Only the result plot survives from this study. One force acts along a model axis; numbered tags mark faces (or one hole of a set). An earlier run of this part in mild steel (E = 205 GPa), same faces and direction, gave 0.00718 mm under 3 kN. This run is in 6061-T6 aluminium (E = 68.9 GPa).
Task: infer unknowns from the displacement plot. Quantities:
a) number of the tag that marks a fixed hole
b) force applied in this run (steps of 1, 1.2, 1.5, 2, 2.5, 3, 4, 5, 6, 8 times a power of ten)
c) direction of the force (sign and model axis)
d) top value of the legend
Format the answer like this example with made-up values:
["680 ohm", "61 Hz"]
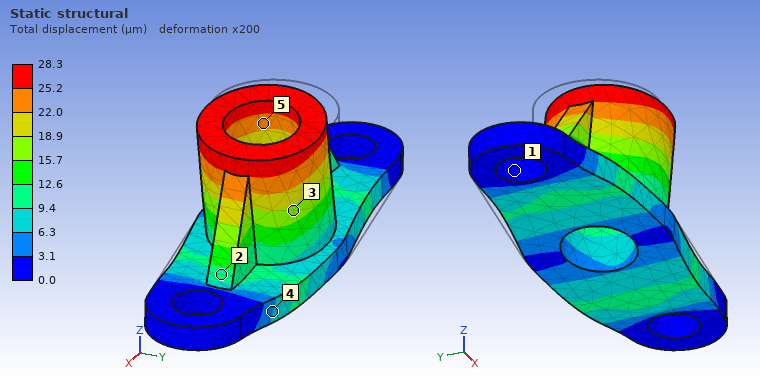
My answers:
["1", "4 kN", "+X", "28.3 µm"]
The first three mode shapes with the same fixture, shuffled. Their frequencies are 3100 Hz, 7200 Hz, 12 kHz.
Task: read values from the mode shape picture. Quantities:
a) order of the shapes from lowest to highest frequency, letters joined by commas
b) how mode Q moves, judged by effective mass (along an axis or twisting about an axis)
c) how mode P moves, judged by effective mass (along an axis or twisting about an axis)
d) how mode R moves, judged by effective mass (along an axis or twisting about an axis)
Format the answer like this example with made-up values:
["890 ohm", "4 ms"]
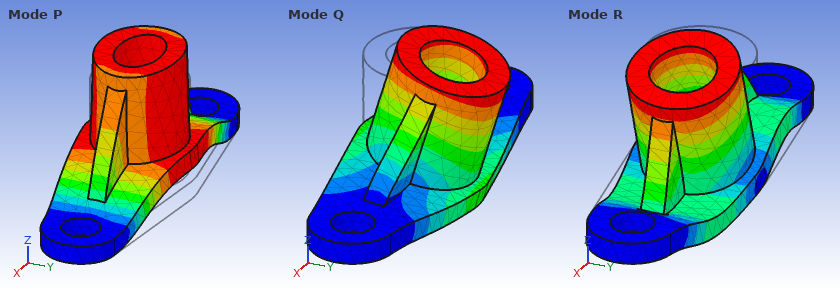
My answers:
["Q, P, R", "along Y", "along Z", "along X"]
